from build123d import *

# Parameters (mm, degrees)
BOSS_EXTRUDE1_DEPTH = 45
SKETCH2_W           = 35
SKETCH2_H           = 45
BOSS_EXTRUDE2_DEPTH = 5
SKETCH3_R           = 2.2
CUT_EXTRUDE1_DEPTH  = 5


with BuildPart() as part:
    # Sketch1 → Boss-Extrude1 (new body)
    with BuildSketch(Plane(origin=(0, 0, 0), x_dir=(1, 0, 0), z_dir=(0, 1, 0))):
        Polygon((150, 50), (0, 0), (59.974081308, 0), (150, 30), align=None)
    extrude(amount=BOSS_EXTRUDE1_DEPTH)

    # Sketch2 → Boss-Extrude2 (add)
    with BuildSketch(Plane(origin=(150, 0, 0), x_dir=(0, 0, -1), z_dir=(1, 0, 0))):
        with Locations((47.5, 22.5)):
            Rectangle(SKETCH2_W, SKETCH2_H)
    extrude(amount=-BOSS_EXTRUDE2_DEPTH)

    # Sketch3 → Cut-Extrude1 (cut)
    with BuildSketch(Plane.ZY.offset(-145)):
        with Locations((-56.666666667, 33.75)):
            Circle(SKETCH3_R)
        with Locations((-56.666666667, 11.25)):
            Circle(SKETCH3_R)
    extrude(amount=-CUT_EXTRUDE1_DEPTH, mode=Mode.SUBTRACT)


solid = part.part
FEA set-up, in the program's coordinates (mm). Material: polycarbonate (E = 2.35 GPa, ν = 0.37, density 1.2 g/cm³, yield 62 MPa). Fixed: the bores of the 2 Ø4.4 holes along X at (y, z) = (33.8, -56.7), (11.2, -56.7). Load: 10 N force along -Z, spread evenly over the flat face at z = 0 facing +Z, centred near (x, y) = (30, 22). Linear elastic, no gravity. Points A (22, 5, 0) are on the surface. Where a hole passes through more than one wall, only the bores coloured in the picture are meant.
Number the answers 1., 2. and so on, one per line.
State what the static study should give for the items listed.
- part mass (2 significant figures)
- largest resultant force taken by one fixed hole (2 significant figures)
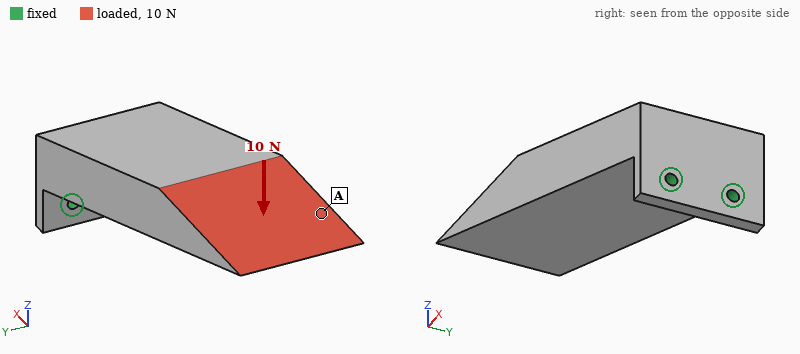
1. 130 g
2. 5.8 N
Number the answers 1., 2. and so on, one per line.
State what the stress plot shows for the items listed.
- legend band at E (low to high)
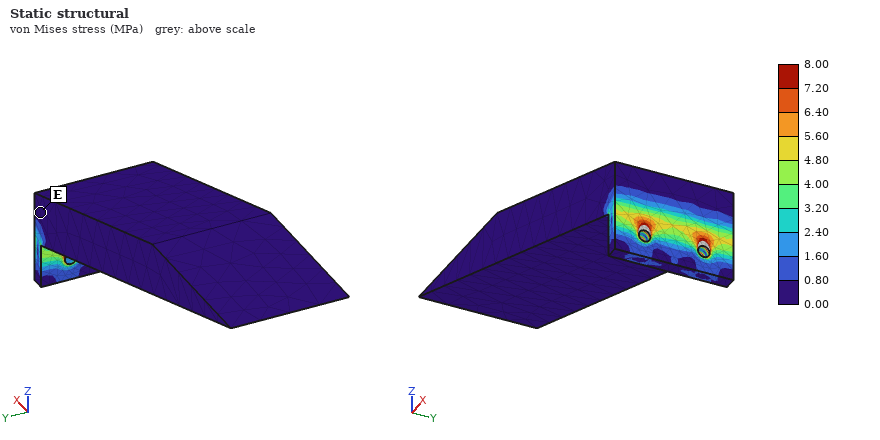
1. 0.00 to 0.80 MPa
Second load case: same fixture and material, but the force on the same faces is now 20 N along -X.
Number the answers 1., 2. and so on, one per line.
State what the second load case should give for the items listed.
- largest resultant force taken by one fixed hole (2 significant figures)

1. 10 N
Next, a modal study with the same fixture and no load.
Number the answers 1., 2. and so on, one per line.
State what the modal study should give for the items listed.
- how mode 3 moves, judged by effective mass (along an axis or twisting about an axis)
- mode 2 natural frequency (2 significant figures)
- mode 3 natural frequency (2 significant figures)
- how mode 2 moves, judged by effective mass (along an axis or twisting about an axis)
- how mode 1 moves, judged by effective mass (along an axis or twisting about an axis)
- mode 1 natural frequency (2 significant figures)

1. along X
2. 170 Hz
3. 770 Hz
4. along Y
5. along Z
6. 57 Hz
